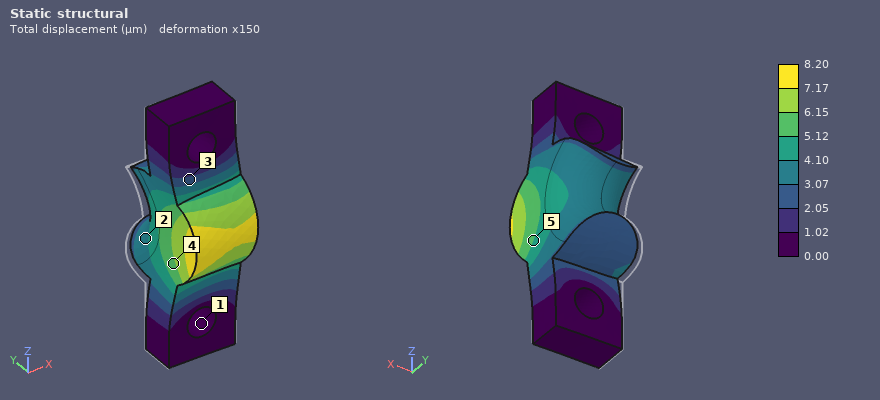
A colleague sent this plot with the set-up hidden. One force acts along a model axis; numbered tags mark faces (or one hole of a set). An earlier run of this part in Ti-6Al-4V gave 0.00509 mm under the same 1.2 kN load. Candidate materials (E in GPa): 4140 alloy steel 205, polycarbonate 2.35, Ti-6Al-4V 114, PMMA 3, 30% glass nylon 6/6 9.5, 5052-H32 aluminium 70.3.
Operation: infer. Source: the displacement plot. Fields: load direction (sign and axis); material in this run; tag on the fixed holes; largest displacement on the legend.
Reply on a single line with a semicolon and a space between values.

+X; 5052-H32 aluminium; 1; 8.20 µm
